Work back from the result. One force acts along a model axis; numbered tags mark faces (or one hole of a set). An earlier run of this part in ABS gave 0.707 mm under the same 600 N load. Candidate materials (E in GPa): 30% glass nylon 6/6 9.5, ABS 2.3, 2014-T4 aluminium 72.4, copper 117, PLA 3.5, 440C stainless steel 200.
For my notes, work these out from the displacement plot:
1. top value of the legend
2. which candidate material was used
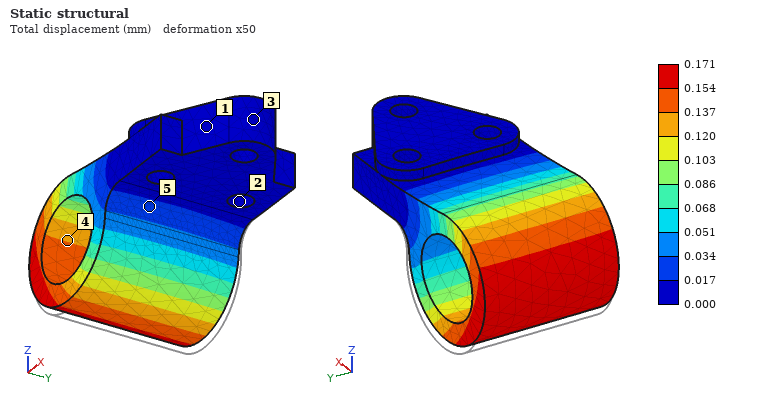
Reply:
0.171 mm
30% glass nylon 6/6
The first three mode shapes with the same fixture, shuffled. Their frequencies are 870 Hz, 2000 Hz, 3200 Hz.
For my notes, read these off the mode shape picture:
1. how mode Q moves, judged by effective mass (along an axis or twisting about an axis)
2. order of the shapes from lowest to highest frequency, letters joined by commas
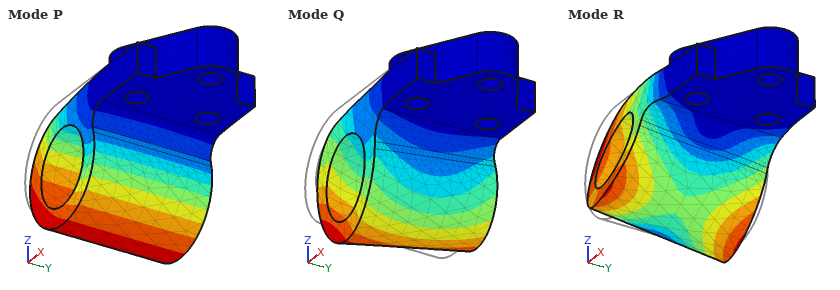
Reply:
along Y
P, Q, R
